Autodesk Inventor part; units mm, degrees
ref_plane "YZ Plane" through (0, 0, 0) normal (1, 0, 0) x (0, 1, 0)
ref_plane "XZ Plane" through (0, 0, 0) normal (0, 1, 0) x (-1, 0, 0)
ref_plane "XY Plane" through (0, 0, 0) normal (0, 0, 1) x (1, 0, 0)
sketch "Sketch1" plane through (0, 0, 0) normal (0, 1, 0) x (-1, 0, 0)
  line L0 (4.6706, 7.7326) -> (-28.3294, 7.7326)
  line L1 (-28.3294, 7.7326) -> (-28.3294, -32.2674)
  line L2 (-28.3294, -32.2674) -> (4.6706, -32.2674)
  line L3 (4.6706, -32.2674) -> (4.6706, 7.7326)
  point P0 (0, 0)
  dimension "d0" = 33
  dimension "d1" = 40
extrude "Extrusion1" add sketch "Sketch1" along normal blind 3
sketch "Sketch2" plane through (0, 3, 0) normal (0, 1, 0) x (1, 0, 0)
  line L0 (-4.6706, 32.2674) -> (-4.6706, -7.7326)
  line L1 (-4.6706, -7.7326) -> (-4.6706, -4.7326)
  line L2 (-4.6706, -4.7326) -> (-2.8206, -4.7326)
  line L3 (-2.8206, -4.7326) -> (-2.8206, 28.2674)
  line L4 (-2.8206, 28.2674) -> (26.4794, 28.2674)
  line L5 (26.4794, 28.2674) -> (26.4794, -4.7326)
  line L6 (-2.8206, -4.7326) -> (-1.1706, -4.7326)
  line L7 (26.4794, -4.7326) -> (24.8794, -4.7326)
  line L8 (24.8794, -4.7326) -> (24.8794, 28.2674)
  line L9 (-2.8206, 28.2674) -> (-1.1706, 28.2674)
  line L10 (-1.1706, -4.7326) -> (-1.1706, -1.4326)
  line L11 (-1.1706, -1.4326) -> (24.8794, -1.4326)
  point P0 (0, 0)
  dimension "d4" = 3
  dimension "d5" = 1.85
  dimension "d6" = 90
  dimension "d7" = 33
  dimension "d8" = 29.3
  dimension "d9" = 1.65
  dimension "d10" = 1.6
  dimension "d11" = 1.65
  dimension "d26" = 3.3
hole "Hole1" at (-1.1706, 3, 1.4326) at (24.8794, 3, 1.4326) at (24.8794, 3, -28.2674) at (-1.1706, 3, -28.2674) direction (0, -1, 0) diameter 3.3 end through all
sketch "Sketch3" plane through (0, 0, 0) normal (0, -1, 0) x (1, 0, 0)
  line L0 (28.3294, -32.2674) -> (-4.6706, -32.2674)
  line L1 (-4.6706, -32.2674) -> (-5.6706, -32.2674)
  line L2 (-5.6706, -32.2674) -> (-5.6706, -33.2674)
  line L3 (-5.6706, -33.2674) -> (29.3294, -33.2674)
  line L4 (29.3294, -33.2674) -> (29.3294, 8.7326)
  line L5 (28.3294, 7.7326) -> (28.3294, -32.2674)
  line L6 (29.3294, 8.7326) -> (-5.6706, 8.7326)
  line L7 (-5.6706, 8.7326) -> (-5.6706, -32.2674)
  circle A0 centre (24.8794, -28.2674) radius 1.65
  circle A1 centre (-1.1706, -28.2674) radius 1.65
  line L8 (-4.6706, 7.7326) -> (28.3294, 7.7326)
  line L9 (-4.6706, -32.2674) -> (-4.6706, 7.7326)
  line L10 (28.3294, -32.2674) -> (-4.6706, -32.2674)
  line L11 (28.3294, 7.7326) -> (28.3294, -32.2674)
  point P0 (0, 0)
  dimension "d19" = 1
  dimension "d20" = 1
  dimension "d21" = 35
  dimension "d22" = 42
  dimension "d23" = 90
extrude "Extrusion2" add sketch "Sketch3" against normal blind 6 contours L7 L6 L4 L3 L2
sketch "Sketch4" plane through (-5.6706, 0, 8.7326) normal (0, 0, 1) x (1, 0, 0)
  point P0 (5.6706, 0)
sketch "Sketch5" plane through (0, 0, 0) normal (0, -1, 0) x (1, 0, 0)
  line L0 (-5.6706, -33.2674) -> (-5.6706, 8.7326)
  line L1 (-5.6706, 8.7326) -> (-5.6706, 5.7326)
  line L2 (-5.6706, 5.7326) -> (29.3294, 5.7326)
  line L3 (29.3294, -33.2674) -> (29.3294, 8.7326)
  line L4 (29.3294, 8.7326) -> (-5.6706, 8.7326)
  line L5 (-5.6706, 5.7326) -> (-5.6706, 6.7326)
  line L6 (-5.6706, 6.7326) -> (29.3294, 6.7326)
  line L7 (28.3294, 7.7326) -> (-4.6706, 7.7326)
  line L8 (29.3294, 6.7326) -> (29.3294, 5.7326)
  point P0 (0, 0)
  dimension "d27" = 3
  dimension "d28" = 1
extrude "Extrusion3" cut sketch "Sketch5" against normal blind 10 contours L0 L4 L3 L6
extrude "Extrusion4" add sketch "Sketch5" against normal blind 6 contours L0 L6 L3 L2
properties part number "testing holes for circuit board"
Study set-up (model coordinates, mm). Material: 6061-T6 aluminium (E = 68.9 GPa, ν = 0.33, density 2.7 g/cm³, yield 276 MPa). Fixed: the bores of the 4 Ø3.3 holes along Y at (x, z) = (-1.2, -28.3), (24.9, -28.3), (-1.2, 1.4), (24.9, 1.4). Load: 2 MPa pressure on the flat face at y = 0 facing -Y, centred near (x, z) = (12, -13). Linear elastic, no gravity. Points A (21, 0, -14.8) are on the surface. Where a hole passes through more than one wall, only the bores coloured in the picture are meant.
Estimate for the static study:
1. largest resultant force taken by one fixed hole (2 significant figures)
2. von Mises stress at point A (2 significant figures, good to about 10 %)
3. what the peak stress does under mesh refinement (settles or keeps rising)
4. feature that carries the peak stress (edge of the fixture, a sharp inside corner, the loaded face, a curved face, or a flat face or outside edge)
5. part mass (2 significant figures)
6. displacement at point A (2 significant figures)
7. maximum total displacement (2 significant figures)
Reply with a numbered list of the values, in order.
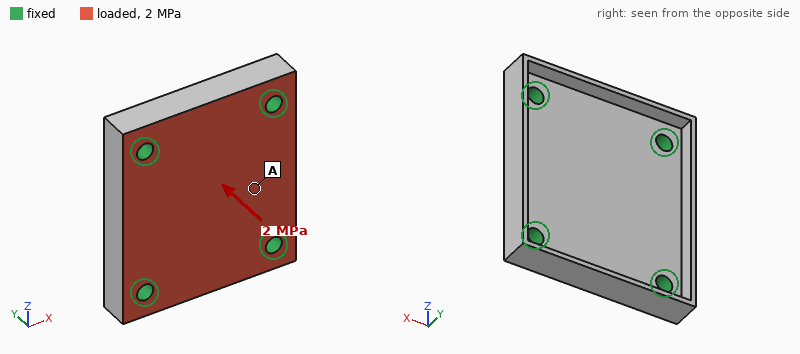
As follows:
1. 690 N
2. 39 MPa
3. keeps rising
4. edge of the fixture
5. 12 g
6. 32 µm
7. 43 µm
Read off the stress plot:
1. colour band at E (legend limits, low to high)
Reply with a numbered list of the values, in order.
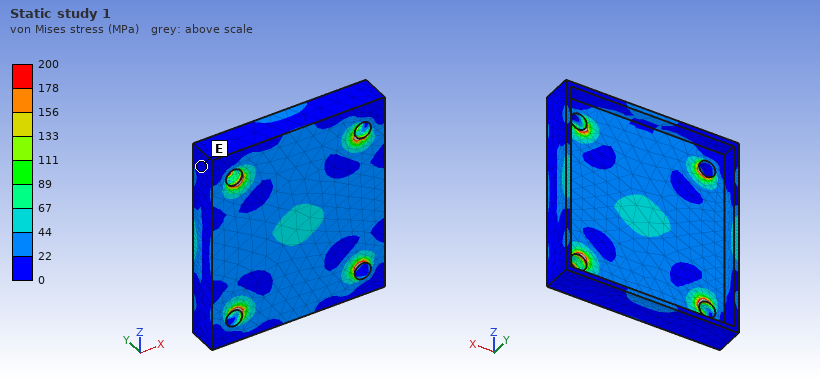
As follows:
1. 0 to 22 MPa
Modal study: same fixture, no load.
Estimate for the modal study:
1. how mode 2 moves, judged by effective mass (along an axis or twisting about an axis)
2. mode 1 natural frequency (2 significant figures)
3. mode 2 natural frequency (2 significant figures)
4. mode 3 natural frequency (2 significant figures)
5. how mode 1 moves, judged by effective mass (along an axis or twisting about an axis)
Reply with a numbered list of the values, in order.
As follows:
1. twisting about Z
2. 15 kHz
3. 22 kHz
4. 24 kHz
5. along Y
